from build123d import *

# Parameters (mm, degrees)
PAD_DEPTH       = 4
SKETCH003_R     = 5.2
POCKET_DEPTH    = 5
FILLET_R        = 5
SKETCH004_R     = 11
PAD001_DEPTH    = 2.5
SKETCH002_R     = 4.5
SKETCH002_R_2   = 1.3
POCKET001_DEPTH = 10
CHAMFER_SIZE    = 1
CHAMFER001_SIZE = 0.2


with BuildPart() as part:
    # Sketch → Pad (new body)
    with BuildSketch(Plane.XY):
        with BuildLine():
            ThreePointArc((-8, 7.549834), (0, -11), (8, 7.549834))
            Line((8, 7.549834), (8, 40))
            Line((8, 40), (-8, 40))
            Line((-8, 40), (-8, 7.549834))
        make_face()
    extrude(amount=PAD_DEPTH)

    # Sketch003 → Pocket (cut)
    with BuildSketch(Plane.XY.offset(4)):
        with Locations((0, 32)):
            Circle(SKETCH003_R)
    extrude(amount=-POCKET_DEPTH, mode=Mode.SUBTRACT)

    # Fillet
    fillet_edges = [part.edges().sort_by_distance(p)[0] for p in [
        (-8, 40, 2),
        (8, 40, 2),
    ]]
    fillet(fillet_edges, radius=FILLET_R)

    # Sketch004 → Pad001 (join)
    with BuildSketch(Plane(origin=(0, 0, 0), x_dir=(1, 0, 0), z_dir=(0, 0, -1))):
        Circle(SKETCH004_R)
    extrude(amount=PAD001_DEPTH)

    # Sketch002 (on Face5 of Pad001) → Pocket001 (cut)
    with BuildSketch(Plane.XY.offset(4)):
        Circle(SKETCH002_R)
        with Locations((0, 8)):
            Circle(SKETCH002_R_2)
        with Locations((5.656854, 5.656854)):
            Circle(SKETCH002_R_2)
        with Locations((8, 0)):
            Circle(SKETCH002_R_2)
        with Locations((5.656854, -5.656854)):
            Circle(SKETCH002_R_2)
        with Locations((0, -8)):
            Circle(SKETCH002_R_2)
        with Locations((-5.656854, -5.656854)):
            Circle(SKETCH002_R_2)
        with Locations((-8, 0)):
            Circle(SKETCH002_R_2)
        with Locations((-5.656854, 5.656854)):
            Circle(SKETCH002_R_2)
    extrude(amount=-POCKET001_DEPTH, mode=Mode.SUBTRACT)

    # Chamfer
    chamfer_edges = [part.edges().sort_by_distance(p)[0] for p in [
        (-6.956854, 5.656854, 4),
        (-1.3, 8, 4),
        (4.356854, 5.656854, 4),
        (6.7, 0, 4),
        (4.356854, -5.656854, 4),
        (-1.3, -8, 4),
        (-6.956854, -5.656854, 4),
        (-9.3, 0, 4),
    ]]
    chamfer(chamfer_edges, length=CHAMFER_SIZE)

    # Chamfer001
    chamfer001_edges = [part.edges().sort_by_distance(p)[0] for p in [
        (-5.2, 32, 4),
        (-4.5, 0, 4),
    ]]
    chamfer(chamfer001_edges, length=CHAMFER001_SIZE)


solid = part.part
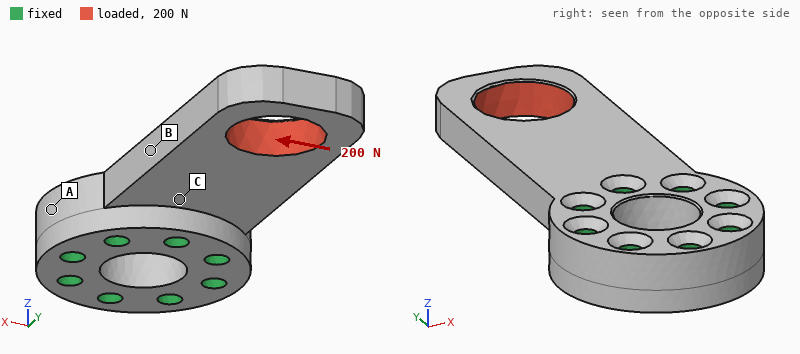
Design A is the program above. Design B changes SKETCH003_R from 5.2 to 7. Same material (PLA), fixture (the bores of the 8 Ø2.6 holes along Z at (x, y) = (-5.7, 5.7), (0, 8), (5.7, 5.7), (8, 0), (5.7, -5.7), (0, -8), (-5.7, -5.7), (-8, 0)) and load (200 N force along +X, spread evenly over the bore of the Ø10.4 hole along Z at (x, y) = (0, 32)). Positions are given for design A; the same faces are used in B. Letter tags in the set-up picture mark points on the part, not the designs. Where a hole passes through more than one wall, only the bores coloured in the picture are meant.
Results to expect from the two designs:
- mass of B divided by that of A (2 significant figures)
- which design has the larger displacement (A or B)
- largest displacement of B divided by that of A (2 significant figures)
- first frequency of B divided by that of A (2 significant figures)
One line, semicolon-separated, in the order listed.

0.92; B; 2.9; 1.2
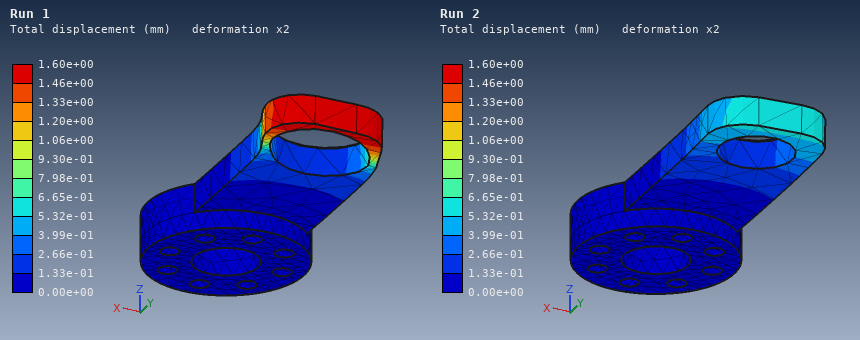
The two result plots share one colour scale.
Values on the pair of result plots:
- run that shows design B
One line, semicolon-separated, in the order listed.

Run 1
